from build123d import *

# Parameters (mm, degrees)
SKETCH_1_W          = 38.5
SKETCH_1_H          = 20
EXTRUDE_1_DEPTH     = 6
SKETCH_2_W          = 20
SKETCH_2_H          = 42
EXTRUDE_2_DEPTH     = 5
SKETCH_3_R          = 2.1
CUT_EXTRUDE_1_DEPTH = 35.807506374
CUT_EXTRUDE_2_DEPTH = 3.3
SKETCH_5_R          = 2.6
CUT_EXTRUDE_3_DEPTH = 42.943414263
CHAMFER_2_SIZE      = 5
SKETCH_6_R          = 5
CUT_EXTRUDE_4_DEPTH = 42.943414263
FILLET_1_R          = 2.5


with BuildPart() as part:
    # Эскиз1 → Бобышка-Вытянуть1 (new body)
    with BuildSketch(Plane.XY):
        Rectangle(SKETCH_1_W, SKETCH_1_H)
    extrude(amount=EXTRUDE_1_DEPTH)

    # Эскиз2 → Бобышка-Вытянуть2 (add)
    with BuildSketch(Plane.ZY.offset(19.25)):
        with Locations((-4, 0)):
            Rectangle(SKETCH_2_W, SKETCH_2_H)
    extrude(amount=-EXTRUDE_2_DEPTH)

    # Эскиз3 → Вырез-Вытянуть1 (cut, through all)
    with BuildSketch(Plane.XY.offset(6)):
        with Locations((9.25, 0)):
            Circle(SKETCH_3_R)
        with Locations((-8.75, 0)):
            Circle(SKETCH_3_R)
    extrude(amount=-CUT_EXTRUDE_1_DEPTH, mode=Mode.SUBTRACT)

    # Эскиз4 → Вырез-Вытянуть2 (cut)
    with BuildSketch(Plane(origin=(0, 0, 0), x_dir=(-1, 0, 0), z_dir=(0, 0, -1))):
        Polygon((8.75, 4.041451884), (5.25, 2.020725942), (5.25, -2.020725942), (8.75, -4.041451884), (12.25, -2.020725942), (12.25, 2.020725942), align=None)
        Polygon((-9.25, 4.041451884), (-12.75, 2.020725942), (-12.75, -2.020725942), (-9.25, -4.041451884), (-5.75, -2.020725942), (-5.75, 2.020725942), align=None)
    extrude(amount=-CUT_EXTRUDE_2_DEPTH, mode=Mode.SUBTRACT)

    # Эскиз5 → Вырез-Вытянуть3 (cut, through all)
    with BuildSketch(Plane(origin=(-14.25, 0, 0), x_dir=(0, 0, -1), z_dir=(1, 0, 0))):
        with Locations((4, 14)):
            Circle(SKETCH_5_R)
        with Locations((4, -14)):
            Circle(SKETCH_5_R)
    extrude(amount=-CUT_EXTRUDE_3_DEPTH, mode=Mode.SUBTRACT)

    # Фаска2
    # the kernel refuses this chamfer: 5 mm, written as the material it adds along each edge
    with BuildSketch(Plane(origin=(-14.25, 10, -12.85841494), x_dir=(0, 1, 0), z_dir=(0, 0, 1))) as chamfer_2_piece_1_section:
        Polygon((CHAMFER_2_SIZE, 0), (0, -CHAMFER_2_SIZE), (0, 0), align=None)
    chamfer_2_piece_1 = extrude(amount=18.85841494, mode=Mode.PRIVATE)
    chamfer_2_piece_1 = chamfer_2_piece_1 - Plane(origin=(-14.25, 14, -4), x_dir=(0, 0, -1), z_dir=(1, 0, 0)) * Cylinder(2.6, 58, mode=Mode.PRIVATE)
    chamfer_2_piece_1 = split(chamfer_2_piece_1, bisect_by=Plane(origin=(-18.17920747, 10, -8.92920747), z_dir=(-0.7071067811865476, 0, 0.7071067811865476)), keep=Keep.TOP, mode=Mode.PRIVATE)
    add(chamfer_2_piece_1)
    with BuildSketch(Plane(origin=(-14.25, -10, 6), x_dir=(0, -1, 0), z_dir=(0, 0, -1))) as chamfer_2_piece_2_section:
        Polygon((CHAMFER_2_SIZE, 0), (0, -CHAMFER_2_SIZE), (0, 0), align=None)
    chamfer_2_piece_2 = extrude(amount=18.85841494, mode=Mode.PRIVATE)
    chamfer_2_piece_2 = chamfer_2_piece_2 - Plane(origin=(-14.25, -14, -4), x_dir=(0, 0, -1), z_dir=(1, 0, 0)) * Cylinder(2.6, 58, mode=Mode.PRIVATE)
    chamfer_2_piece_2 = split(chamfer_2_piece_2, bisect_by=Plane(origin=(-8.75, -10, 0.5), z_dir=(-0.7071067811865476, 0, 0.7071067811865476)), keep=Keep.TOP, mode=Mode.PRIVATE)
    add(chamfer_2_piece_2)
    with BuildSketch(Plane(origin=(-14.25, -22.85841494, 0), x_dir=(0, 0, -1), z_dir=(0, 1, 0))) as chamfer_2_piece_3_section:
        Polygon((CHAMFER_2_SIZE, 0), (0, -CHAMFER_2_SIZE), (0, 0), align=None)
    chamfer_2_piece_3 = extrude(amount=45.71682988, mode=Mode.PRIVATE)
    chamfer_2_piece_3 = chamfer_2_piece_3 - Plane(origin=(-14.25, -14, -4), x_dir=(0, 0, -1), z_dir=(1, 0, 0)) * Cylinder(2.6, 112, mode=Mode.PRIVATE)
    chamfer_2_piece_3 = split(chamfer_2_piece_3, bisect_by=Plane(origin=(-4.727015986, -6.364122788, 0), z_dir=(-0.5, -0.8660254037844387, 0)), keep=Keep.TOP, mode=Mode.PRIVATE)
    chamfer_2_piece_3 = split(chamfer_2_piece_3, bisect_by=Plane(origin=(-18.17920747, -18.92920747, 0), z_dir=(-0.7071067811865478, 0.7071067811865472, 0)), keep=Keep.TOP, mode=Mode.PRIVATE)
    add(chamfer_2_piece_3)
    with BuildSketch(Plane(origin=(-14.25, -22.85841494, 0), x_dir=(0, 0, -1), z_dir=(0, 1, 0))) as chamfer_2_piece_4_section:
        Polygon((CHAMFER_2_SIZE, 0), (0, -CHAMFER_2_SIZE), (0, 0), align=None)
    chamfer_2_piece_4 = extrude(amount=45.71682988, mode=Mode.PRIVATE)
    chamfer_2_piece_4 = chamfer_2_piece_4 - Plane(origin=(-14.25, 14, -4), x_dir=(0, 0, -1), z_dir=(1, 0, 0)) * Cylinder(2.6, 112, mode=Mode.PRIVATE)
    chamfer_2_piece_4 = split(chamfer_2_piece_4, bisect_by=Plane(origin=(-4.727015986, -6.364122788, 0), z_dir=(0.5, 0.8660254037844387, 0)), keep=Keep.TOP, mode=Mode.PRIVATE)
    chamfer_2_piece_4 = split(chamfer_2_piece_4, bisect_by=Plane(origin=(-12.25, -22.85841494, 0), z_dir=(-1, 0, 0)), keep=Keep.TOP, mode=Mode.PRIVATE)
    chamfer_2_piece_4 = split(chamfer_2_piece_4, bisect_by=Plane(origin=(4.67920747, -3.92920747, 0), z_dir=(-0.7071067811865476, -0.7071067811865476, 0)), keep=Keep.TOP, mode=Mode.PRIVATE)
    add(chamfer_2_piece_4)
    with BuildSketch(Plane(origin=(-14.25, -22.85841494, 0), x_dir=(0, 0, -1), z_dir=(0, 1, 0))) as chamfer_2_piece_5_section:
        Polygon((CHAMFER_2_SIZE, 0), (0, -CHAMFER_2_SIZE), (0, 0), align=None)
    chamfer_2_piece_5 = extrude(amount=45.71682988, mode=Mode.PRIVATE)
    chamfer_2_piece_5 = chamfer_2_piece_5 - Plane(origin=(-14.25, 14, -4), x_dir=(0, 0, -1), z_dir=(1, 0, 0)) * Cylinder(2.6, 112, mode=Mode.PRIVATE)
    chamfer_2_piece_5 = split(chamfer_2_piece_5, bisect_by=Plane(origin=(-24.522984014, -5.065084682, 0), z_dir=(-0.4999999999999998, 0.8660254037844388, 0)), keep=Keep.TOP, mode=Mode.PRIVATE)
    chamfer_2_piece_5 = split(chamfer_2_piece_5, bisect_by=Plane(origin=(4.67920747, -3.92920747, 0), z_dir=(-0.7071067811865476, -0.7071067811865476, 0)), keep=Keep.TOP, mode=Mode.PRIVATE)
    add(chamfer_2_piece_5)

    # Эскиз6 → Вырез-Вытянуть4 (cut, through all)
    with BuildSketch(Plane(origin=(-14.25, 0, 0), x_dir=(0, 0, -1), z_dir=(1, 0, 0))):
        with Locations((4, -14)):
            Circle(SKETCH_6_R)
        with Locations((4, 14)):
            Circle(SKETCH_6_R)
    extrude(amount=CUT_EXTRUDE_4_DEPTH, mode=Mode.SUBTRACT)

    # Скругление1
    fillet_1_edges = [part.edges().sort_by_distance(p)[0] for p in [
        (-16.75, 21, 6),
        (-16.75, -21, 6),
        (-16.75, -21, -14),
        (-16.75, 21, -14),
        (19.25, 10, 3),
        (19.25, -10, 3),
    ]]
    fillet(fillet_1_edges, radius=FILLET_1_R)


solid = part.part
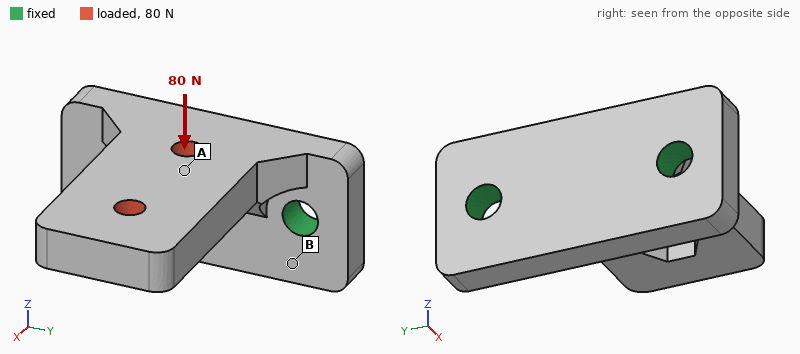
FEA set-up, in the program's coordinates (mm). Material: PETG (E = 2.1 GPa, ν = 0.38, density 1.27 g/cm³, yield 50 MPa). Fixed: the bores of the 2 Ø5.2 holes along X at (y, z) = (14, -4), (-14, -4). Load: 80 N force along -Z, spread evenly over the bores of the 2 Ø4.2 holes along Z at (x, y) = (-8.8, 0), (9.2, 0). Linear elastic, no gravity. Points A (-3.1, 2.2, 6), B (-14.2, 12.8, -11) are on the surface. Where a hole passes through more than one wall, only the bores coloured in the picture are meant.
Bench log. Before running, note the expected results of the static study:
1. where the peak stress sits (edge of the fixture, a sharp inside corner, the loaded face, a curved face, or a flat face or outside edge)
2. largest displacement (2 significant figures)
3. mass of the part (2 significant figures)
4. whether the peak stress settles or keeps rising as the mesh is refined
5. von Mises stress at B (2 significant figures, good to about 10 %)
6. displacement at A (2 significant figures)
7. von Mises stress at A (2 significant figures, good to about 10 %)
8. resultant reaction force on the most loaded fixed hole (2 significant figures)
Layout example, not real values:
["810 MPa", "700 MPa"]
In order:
["a sharp inside corner", "0.69 mm", "10 g", "keeps rising", "1.7 MPa", "0.20 mm", "3.9 MPa", "40 N"]
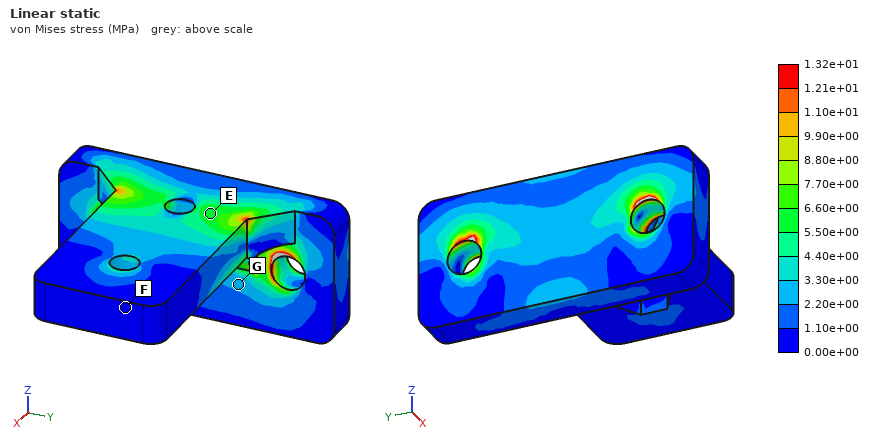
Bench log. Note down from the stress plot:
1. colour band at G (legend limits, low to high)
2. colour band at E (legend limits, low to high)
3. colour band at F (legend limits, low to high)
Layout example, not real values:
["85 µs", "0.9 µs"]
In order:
["2.20e+00 to 3.30e+00 MPa", "5.50e+00 to 6.60e+00 MPa", "0.00e+00 to 1.10e+00 MPa"]
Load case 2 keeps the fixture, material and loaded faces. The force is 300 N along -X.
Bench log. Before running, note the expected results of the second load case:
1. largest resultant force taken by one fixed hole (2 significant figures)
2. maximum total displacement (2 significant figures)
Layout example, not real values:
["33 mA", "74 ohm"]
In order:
["160 N", "0.66 mm"]
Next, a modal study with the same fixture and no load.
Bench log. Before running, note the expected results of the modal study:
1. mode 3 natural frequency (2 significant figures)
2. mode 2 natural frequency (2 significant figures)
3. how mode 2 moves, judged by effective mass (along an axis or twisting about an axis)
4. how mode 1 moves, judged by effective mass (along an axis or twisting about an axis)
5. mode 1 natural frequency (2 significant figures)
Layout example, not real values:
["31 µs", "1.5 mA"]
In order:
["3300 Hz", "2400 Hz", "along Y", "along Z", "900 Hz"]
